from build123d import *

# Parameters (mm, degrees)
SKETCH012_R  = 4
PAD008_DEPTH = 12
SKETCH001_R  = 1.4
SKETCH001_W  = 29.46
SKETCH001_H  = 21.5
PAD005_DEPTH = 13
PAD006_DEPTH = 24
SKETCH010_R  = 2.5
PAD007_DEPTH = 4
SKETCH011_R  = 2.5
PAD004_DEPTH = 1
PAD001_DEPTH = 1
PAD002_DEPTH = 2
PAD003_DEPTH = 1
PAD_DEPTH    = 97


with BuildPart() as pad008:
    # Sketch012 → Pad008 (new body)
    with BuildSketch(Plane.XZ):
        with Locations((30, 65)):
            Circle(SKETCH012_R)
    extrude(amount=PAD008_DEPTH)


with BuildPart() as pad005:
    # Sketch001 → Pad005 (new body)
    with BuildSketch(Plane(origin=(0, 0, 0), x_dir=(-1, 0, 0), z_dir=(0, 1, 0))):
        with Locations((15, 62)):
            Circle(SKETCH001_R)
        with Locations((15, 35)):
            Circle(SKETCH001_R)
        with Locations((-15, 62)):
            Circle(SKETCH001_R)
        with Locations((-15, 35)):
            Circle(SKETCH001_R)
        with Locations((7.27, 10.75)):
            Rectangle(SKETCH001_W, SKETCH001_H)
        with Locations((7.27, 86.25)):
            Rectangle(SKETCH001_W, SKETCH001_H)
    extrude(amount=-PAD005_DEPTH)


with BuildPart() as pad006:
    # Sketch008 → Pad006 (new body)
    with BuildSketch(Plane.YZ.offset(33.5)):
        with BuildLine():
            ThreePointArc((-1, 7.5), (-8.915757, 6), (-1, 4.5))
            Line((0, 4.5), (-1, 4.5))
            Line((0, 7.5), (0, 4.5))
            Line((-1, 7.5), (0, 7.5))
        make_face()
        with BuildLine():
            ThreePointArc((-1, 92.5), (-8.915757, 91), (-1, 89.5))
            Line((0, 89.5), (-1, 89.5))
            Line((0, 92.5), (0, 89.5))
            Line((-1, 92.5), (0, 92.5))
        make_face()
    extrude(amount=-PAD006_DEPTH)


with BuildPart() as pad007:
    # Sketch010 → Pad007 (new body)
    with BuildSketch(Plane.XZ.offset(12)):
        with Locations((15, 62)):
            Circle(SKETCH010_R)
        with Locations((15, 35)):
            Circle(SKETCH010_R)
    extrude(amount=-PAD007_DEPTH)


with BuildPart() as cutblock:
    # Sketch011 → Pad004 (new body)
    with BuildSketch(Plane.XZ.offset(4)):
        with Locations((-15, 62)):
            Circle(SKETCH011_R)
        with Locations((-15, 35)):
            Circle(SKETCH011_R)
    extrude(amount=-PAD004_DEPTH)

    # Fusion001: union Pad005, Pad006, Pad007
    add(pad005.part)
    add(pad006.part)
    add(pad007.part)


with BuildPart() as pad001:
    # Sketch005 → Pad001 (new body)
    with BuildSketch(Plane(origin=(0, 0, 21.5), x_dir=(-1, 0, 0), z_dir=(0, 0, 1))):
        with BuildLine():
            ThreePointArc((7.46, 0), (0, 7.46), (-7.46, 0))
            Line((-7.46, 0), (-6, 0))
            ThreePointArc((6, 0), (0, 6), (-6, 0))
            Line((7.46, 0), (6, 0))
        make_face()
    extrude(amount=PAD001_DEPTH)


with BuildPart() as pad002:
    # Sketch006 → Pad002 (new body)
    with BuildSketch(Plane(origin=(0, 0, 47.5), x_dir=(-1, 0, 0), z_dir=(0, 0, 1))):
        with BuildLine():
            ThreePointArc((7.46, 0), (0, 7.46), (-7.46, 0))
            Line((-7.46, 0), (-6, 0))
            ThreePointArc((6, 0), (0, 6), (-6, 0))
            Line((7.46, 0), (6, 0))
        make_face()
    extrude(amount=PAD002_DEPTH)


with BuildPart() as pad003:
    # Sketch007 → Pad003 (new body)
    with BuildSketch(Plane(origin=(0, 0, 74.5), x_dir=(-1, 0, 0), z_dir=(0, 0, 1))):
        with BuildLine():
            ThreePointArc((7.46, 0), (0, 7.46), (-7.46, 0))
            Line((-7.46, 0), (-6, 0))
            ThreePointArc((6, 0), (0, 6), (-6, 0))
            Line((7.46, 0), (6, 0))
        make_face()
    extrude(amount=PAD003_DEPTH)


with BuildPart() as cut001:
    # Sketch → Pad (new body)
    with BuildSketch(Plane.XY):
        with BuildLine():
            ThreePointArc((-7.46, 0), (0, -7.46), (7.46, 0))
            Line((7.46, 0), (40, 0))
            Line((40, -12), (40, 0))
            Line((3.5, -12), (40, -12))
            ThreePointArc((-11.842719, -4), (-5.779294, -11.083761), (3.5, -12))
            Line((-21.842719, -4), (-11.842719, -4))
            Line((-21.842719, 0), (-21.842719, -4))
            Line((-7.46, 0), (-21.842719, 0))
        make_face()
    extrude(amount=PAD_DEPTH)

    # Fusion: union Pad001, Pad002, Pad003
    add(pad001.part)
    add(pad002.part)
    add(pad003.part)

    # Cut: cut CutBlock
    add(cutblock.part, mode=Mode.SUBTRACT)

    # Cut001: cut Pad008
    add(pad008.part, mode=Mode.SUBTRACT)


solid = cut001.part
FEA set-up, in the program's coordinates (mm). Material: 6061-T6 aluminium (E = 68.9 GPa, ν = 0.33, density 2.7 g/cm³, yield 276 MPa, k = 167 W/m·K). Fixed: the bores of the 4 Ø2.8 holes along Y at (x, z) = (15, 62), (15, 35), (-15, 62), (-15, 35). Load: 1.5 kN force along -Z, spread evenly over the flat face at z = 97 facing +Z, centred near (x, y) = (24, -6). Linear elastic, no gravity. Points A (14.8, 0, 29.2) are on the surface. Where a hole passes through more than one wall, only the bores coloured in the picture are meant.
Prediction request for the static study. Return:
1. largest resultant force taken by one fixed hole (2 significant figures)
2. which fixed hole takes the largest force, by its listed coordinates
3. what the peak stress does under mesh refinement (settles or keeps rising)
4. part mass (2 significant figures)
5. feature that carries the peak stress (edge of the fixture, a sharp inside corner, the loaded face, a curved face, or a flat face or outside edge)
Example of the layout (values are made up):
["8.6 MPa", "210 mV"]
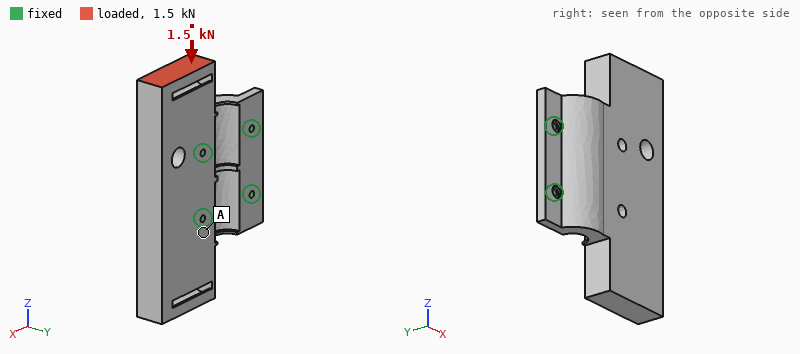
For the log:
["1.1 kN", "(15, 62)", "keeps rising", "120 g", "a sharp inside corner"]
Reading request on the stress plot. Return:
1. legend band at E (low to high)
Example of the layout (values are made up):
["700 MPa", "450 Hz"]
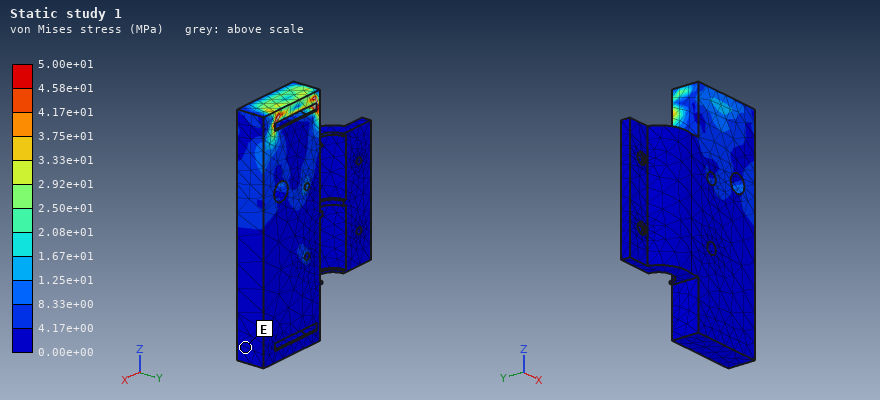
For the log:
["0.00e+00 to 4.17e+00 MPa"]
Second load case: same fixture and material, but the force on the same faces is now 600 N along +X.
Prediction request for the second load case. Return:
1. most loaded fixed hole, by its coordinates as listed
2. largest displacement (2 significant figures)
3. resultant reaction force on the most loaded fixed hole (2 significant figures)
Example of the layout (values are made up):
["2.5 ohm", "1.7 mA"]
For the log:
["(15, 62)", "17 µm", "970 N"]
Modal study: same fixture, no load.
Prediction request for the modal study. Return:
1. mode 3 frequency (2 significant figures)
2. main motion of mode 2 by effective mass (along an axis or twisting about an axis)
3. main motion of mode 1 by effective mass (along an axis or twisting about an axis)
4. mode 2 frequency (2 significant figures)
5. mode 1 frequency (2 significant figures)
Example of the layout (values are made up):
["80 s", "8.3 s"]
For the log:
["8300 Hz", "along Y", "twisting about X", "5600 Hz", "5200 Hz"]
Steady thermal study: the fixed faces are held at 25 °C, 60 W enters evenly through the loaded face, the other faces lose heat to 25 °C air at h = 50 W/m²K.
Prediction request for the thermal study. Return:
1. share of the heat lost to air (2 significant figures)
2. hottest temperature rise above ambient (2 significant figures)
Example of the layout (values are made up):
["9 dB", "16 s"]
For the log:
["11 %", "59 K"]
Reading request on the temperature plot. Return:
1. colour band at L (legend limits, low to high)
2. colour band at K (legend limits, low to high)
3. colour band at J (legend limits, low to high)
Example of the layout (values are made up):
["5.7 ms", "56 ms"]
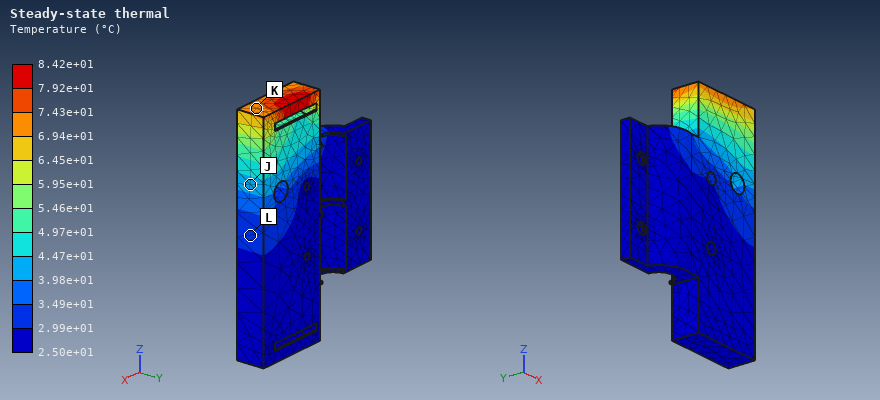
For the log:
["2.99e+01 to 3.49e+01 °C", "6.94e+01 to 7.43e+01 °C", "3.98e+01 to 4.47e+01 °C"]
